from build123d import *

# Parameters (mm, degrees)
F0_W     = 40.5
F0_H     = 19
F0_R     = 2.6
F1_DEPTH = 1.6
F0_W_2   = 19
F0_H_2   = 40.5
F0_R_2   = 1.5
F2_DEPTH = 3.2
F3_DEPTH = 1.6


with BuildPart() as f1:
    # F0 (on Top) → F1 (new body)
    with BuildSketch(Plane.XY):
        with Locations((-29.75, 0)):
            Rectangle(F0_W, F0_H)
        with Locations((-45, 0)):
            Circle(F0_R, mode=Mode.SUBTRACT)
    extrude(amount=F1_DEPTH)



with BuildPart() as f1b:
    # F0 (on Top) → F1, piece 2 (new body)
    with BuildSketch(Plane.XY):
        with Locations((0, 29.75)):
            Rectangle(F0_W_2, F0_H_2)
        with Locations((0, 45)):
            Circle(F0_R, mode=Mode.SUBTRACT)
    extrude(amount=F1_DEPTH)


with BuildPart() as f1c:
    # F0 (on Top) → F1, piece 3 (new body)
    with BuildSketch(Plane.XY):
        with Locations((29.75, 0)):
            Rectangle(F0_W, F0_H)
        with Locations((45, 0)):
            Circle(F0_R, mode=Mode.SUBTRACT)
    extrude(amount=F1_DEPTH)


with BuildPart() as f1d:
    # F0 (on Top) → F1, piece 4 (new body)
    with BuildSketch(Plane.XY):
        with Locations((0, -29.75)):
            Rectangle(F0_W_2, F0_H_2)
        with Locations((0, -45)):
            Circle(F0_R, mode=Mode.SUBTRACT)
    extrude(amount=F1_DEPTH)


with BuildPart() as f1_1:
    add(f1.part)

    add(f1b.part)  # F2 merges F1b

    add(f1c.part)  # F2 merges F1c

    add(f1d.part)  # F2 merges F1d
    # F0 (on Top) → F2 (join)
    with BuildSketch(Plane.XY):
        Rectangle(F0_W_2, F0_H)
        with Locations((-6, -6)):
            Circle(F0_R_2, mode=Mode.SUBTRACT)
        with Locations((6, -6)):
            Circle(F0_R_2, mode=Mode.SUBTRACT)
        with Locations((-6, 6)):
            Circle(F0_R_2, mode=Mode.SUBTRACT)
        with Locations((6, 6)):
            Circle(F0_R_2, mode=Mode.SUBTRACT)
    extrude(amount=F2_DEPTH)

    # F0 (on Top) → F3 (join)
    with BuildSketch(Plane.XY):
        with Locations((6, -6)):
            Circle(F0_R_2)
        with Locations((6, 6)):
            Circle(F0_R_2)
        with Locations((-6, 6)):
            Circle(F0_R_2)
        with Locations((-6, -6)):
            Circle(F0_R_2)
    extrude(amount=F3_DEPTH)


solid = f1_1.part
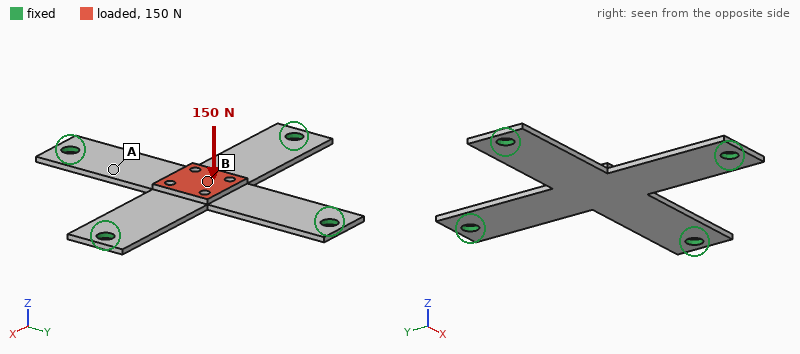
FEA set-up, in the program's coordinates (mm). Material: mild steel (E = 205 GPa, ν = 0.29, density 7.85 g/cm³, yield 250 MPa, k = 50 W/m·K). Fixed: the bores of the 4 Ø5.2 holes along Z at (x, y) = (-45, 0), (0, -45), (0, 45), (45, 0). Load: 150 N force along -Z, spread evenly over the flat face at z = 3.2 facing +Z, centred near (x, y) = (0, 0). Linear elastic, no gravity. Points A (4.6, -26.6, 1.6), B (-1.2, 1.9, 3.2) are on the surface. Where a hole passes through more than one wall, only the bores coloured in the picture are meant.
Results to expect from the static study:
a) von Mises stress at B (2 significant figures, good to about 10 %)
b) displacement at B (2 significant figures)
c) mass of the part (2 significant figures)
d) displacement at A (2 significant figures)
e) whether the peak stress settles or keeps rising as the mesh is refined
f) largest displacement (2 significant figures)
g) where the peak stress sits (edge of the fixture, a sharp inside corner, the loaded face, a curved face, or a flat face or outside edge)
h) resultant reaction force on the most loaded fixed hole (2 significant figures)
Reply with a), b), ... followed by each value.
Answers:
a) 23 MPa
b) 0.10 mm
c) 46 g
d) 0.048 mm
e) keeps rising
f) 0.10 mm
g) edge of the fixture
h) 53 N
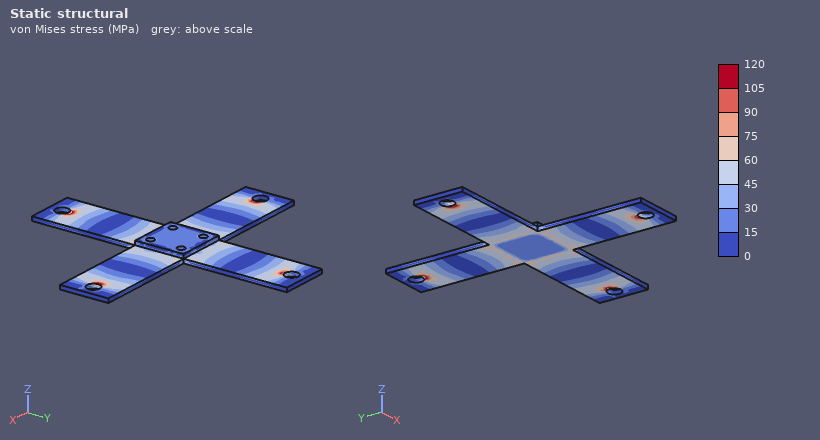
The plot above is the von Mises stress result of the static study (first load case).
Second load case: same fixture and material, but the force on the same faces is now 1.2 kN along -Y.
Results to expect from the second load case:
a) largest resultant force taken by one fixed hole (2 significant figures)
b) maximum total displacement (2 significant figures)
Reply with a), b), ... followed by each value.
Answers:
a) 560 N
b) 49 µm
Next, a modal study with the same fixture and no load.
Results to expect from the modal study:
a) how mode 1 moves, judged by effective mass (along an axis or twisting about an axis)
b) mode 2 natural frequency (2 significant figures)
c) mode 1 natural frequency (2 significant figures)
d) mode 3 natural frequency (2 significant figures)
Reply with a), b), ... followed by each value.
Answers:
a) along Z
b) 3200 Hz
c) 1400 Hz
d) 3200 Hz
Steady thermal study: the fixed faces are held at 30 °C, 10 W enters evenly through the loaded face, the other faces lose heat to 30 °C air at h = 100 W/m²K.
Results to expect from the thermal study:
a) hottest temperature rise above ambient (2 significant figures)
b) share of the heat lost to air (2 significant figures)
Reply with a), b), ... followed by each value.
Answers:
a) 32 K
b) 75 %
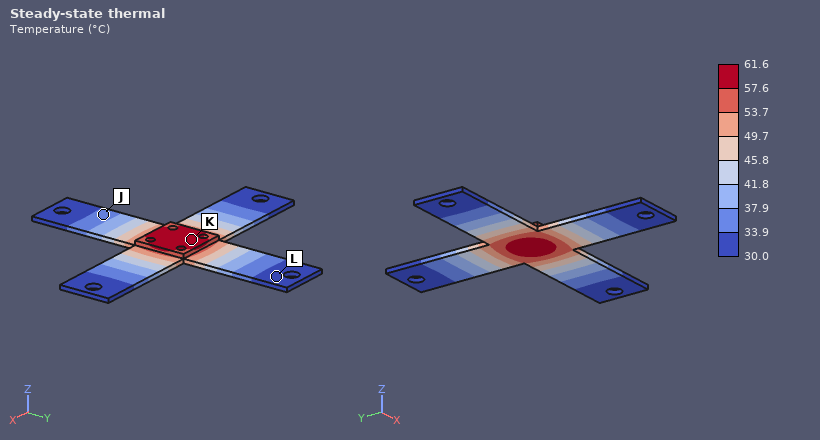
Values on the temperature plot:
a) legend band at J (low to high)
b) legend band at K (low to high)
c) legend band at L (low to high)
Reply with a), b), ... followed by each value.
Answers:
a) 33.9 to 37.9 °C
b) 57.6 to 61.6 °C
c) 30.0 to 33.9 °C
